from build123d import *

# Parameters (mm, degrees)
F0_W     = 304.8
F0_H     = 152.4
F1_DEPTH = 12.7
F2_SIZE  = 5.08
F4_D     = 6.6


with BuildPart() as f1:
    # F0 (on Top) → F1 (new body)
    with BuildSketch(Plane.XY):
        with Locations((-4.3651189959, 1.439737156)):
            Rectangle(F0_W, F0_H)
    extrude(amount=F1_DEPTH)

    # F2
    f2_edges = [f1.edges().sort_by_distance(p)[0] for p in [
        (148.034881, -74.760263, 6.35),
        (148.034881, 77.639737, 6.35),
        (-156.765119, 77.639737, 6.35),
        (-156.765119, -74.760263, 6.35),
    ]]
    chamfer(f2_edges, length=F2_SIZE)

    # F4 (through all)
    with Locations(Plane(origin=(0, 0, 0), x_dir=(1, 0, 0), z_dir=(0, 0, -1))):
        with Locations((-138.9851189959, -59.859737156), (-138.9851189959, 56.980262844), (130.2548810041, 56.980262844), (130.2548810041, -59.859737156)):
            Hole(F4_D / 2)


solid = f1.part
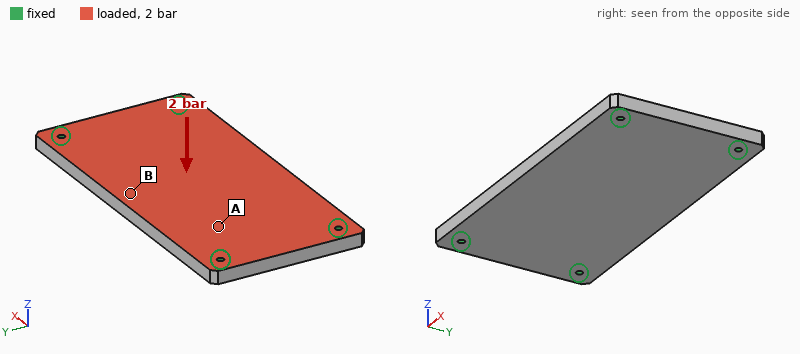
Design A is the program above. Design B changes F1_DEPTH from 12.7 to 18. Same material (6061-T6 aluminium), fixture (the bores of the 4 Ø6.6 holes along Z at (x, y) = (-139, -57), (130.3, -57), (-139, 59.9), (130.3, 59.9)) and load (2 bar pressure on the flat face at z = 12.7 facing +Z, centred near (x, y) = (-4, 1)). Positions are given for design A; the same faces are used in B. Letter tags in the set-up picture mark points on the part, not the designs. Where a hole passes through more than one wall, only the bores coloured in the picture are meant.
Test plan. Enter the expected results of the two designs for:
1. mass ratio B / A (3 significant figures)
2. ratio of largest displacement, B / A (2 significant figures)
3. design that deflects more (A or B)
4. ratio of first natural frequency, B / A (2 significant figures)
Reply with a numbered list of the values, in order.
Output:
1. 1.42
2. 0.38
3. A
4. 1.4
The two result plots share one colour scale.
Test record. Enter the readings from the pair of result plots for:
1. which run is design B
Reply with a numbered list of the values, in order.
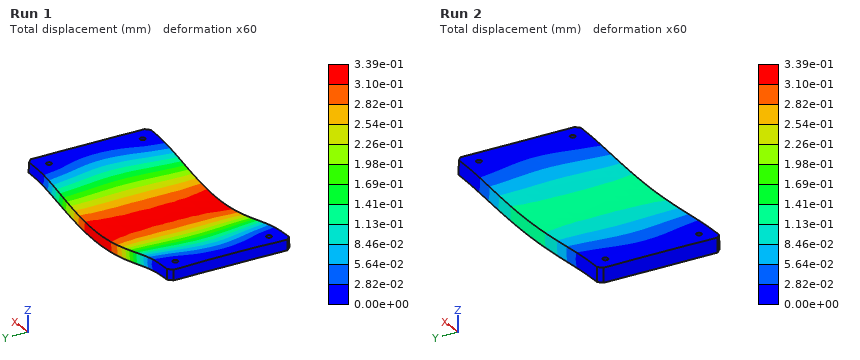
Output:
1. Run 2
